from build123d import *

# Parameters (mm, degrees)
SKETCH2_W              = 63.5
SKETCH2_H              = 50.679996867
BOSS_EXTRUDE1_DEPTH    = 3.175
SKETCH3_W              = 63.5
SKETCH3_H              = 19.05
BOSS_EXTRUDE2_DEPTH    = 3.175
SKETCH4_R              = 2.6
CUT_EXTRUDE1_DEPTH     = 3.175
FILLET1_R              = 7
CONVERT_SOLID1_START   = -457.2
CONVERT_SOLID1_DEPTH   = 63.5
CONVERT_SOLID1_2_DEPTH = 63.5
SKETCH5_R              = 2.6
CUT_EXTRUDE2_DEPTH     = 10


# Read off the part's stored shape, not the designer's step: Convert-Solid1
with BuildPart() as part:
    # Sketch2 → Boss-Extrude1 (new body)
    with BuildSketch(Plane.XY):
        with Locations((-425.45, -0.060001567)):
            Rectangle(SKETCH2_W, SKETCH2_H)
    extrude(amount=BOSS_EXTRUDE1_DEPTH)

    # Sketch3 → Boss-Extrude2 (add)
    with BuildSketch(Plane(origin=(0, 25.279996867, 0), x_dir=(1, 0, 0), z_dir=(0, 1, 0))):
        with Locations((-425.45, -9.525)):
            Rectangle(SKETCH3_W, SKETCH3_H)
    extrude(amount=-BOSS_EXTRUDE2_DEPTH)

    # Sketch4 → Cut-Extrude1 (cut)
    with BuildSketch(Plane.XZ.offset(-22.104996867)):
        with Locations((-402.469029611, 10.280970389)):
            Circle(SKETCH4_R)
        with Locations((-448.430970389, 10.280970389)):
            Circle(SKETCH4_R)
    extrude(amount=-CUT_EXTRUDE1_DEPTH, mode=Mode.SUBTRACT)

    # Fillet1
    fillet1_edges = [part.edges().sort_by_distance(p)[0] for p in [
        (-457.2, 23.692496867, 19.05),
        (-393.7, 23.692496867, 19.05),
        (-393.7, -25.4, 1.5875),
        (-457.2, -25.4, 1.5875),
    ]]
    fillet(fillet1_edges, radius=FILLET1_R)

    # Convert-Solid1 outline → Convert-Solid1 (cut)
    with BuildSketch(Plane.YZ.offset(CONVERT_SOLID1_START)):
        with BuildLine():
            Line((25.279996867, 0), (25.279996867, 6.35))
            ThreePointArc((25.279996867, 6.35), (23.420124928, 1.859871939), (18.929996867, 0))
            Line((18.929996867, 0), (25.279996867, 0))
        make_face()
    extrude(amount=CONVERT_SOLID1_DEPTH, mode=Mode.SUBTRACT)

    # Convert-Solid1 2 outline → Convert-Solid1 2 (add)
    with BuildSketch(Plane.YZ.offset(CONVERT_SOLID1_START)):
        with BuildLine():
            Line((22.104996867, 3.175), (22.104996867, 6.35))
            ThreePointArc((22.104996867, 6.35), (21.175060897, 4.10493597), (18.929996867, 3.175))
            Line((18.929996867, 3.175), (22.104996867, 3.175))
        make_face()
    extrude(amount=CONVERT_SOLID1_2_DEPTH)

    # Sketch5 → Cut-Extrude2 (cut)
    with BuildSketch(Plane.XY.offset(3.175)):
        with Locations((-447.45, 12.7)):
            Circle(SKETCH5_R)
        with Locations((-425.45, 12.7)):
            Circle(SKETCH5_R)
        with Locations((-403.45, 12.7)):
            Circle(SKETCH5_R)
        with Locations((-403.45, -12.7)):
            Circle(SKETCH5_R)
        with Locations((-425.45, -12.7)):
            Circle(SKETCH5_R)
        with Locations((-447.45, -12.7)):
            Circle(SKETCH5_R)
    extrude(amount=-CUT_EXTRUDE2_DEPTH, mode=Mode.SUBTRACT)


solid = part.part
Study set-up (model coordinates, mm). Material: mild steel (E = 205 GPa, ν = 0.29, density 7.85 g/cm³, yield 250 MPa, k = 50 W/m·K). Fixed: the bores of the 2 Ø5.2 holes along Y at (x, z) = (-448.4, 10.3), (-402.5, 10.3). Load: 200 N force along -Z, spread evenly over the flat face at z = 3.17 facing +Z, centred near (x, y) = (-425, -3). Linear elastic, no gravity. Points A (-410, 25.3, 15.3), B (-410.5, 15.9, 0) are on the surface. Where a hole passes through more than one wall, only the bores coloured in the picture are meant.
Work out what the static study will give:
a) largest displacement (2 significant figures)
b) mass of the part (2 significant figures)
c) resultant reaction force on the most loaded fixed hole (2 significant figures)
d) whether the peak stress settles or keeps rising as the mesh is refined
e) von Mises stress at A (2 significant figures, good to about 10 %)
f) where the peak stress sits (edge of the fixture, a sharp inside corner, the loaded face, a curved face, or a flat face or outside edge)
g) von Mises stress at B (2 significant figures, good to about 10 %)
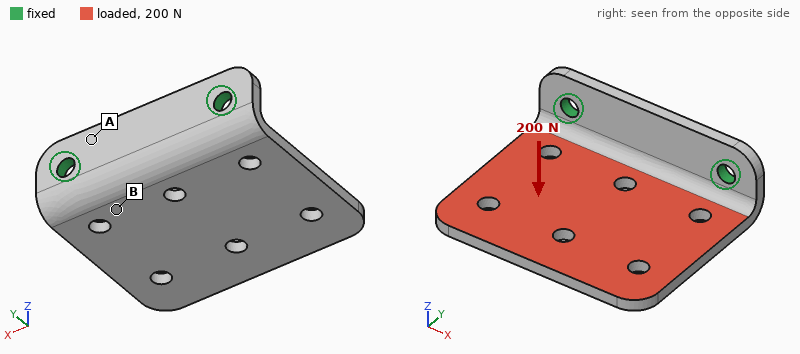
0.16 mm
97 g
100 N
keeps rising
14 MPa
edge of the fixture
38 MPa
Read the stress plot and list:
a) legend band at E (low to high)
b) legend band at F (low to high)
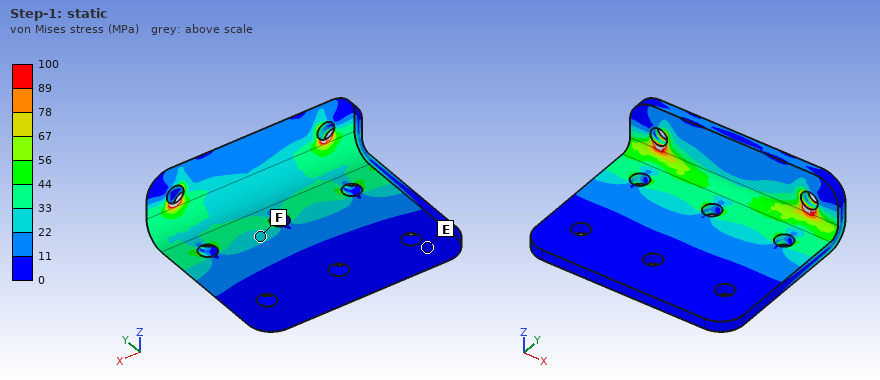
0 to 11 MPa
22 to 33 MPa
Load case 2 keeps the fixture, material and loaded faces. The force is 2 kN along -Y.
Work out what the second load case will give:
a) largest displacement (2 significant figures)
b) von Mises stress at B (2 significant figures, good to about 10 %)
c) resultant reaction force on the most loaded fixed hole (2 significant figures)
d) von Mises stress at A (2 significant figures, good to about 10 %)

24 µm
20 MPa
1.0 kN
20 MPa
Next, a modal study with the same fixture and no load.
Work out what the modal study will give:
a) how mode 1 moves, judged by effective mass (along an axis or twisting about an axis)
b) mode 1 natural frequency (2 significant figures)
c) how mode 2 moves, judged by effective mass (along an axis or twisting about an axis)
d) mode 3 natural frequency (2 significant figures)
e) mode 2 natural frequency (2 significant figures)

along Z
860 Hz
twisting about Y
5000 Hz
2000 Hz
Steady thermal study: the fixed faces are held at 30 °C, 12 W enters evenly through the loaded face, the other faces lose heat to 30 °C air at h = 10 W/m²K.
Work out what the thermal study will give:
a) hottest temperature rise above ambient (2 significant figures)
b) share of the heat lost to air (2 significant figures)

43 K
12 %
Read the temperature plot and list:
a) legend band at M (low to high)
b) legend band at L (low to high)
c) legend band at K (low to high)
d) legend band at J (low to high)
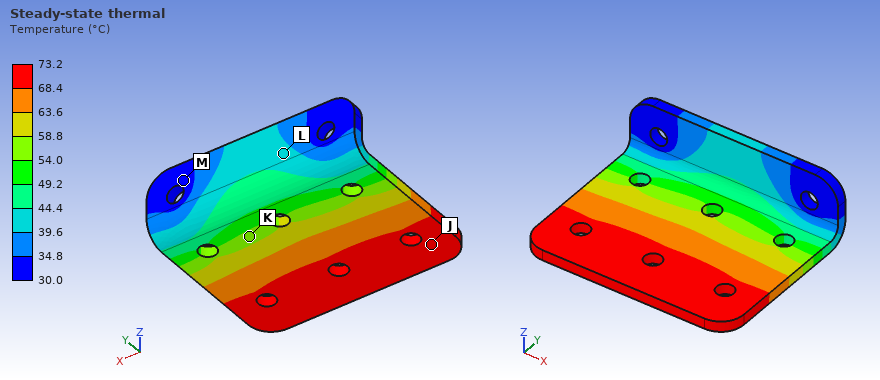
30.0 to 34.8 °C
39.6 to 44.4 °C
54.0 to 58.8 °C
68.4 to 73.2 °C
